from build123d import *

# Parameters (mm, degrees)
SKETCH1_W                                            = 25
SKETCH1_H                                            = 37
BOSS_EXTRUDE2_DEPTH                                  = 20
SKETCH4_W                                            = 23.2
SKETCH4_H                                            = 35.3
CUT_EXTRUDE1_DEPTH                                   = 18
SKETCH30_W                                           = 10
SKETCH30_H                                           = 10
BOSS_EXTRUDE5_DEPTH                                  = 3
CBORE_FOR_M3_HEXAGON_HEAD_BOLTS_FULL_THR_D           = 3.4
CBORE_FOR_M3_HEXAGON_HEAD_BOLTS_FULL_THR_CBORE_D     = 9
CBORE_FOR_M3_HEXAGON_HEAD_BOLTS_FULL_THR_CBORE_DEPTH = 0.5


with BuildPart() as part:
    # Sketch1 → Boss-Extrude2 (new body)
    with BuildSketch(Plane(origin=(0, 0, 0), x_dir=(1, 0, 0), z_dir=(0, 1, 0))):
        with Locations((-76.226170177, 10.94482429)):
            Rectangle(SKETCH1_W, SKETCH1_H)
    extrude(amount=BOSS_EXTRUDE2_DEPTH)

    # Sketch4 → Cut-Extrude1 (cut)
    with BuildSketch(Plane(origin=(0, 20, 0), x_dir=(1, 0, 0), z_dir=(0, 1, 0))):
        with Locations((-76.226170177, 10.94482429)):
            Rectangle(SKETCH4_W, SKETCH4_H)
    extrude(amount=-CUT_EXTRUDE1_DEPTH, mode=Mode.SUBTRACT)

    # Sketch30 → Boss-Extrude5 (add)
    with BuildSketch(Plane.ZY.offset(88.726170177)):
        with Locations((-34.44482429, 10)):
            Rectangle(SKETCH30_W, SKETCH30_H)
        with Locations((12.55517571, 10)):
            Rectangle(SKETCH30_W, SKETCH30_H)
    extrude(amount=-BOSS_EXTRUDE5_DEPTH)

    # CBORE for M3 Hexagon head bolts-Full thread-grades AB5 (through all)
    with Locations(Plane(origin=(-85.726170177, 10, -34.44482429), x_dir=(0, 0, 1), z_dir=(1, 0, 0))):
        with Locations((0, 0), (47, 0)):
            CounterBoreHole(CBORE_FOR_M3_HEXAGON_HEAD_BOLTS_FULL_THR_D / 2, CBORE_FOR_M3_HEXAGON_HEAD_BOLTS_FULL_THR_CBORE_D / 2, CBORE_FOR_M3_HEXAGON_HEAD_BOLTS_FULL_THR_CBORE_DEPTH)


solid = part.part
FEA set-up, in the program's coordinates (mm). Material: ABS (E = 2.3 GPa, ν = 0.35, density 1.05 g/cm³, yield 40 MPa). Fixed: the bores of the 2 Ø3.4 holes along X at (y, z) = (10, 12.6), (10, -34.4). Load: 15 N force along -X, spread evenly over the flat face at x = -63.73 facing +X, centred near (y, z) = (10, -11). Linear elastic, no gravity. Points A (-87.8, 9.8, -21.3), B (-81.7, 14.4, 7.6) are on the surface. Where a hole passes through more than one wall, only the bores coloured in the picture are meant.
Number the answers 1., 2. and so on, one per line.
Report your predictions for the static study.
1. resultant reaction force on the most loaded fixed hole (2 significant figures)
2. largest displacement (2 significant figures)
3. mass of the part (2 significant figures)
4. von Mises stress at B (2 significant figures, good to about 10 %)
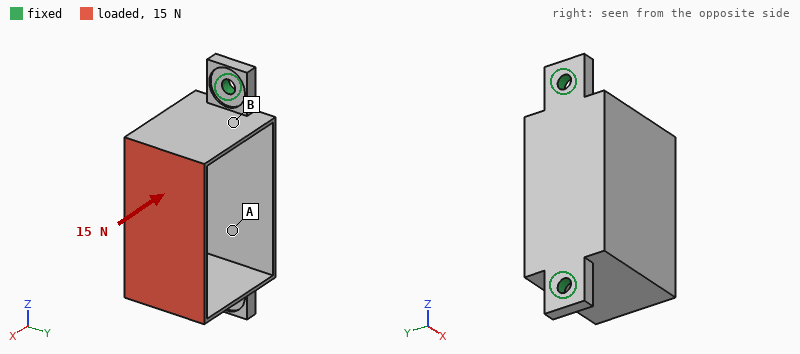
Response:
1. 7.6 N
2. 0.66 mm
3. 4.5 g
4. 1.8 MPa
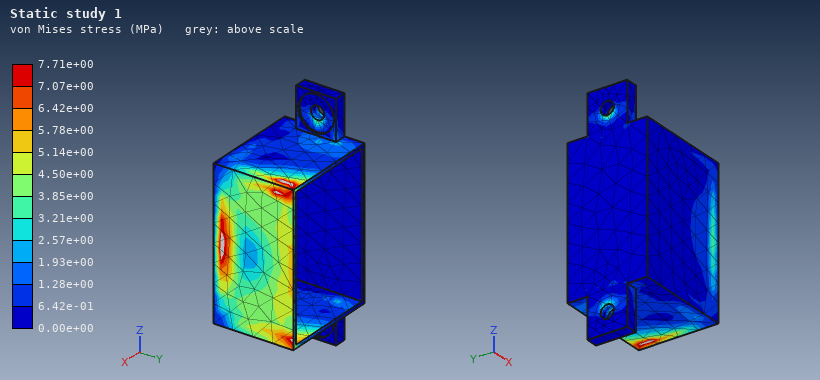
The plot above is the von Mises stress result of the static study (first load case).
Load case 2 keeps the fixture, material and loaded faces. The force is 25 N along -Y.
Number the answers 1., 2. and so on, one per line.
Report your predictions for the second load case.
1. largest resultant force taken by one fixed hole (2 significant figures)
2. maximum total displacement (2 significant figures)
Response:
1. 13 N
2. 0.78 mm
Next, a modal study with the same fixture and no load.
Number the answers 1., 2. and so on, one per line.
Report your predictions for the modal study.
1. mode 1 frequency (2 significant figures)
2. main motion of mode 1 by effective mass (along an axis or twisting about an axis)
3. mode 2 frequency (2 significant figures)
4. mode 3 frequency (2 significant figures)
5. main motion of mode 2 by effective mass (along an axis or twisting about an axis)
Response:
1. 710 Hz
2. along Y
3. 840 Hz
4. 1200 Hz
5. along Z
